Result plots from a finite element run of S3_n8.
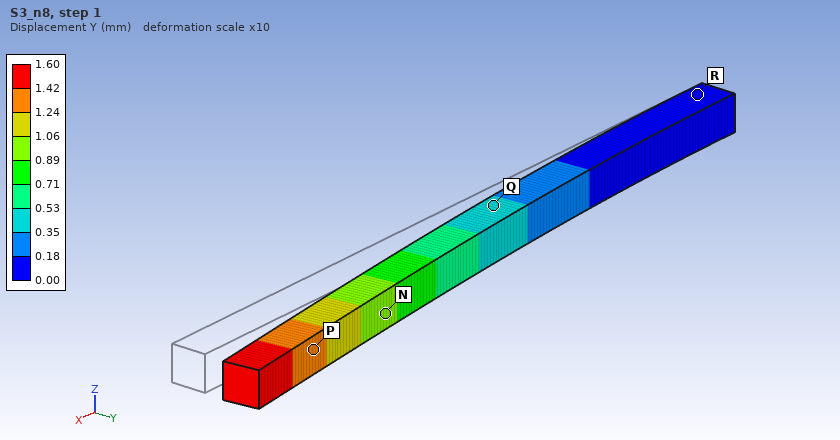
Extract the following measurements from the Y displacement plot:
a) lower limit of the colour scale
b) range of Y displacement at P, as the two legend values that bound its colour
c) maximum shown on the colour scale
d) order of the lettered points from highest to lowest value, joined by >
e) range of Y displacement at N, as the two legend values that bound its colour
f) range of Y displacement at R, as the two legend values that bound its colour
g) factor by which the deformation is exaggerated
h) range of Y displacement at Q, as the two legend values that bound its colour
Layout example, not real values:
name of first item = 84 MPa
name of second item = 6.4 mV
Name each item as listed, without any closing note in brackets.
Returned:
lower limit of the colour scale = 0.00 mm
range of Y displacement at P, as the two legend values that bound its colour = 1.24 to 1.42 mm
maximum shown on the colour scale = 1.60 mm
order of the lettered points from highest to lowest value, joined by > = P > N > Q > R
range of Y displacement at N, as the two legend values that bound its colour = 0.89 to 1.06 mm
range of Y displacement at R, as the two legend values that bound its colour = 0.00 to 0.18 mm
factor by which the deformation is exaggerated = 10
range of Y displacement at Q, as the two legend values that bound its colour = 0.35 to 0.53 mm
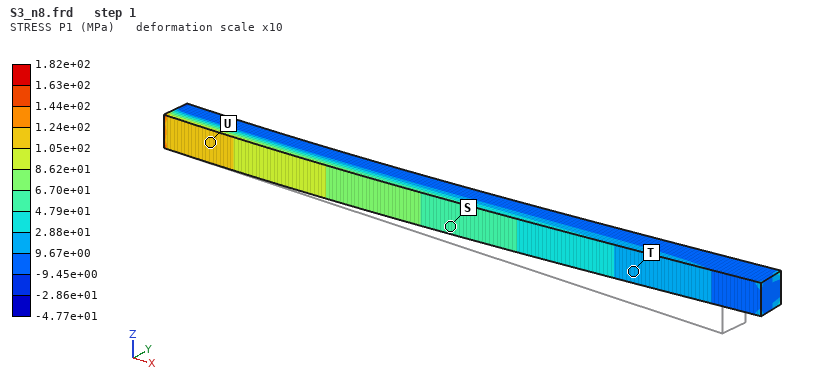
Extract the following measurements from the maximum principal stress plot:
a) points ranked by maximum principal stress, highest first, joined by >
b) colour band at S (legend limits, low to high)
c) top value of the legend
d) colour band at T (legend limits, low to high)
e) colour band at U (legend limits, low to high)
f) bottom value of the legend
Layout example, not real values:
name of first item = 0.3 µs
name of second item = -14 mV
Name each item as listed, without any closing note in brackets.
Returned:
points ranked by maximum principal stress, highest first, joined by > = U > S > T
colour band at S = 4.79e+01 to 6.70e+01 MPa
top value of the legend = 1.82e+02 MPa
colour band at T = 9.67e+00 to 2.88e+01 MPa
colour band at U = 1.05e+02 to 1.24e+02 MPa
bottom value of the legend = -4.77e+01 MPa
